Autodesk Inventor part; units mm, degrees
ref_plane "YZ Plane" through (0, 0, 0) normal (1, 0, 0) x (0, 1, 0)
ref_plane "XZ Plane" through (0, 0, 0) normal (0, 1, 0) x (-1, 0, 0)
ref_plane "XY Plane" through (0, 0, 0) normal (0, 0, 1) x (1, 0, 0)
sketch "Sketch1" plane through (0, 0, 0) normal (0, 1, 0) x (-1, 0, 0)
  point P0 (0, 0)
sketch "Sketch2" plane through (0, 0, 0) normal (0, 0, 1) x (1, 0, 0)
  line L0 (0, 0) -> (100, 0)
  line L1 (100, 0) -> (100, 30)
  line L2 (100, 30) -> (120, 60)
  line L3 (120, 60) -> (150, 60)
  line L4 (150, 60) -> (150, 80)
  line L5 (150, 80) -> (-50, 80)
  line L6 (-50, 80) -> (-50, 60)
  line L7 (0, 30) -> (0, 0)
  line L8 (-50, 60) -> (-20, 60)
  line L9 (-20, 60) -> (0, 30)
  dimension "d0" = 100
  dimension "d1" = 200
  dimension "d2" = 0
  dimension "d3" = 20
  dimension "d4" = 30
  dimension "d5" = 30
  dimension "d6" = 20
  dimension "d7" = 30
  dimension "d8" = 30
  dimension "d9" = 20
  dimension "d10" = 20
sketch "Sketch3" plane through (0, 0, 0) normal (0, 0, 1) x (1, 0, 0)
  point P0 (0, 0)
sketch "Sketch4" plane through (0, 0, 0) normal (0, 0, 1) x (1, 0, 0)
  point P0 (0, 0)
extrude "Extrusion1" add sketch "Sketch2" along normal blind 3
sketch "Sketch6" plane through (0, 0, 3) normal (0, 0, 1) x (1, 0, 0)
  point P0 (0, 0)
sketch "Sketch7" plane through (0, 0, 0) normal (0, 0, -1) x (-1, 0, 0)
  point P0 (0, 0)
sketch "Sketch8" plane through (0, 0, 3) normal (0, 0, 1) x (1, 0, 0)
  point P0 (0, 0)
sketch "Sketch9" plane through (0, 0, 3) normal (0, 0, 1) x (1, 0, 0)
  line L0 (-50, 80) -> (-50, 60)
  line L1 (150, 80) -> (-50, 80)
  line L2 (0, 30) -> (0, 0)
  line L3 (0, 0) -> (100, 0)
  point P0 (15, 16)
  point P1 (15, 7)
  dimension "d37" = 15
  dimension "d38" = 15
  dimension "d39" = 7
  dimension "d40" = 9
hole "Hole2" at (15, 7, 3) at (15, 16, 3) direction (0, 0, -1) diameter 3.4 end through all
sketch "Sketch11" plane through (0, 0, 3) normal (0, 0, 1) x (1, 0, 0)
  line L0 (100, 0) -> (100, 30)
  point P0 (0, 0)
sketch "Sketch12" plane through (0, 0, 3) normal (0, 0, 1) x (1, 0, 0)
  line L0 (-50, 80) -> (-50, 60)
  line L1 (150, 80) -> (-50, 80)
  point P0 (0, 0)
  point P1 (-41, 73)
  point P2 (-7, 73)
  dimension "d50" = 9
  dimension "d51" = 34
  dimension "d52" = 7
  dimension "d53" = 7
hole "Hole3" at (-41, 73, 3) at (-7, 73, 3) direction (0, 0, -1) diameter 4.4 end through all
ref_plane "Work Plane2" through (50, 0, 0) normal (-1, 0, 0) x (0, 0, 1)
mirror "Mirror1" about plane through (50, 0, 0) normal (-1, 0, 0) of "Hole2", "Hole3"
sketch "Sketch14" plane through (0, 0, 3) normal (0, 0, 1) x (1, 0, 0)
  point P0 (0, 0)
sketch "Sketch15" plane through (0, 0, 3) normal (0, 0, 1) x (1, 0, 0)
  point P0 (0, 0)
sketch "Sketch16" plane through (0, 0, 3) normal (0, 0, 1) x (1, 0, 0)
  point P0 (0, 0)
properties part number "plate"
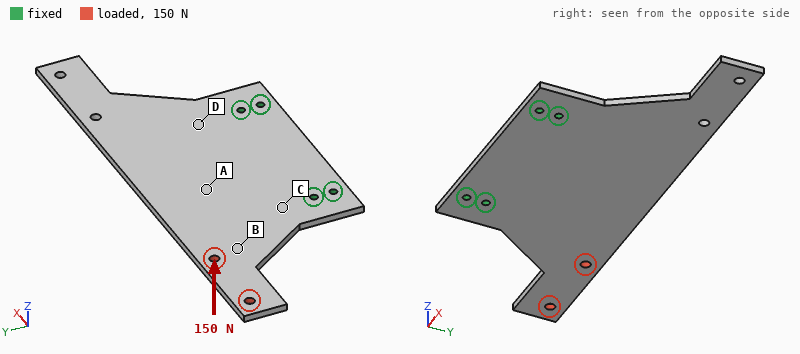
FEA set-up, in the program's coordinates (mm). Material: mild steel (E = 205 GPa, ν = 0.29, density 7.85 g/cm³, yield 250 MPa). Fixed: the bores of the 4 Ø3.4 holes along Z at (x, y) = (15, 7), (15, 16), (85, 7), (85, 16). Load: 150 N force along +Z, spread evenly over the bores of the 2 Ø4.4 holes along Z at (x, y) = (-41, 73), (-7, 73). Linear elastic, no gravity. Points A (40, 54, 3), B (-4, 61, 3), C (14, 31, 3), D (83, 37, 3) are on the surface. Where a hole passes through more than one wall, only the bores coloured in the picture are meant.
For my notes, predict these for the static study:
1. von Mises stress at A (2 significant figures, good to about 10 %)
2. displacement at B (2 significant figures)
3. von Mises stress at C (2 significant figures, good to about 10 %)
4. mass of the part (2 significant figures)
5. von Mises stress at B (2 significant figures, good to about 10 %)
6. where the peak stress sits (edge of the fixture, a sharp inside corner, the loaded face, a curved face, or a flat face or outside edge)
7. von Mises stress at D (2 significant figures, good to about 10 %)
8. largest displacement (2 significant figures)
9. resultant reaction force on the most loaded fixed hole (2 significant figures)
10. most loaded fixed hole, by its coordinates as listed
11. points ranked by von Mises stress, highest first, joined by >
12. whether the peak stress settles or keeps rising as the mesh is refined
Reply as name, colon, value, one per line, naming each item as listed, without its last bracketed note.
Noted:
von Mises stress at A: 49 MPa
displacement at B: 0.41 mm
von Mises stress at C: 91 MPa
mass of the part: 250 g
von Mises stress at B: 71 MPa
where the peak stress sits: edge of the fixture
von Mises stress at D: 19 MPa
largest displacement: 1.2 mm
resultant reaction force on the most loaded fixed hole: 560 N
most loaded fixed hole, by its coordinates as listed: (15, 16)
points ranked by von Mises stress, highest first, joined by >: C > B > A > D
whether the peak stress settles or keeps rising as the mesh is refined: keeps rising
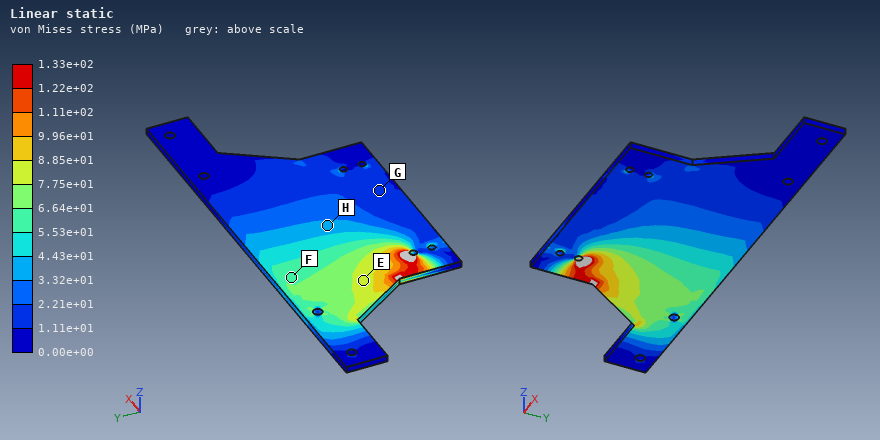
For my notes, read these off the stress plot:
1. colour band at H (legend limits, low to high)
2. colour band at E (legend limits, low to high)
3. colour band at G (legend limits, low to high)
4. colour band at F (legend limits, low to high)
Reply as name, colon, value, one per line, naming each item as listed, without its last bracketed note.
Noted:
colour band at H: 3.32e+01 to 4.43e+01 MPa
colour band at E: 7.75e+01 to 8.85e+01 MPa
colour band at G: 1.11e+01 to 2.21e+01 MPa
colour band at F: 5.53e+01 to 6.64e+01 MPa
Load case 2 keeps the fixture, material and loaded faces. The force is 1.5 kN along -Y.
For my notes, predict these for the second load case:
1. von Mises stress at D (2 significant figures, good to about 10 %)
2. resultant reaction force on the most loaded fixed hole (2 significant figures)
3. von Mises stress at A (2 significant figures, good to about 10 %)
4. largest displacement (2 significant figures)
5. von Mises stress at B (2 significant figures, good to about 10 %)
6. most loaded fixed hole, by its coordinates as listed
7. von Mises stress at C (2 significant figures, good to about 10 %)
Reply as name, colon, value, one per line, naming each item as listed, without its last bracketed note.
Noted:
von Mises stress at D: 8.3 MPa
resultant reaction force on the most loaded fixed hole: 1.6 kN
von Mises stress at A: 12 MPa
largest displacement: 66 µm
von Mises stress at B: 16 MPa
most loaded fixed hole, by its coordinates as listed: (15, 16)
von Mises stress at C: 24 MPa
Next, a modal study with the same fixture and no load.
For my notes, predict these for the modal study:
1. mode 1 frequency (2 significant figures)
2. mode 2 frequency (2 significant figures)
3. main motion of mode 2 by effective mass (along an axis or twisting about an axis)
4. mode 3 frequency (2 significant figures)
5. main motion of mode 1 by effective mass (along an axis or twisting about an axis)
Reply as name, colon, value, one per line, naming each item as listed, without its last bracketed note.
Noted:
mode 1 frequency: 380 Hz
mode 2 frequency: 420 Hz
main motion of mode 2 by effective mass: twisting about Y
mode 3 frequency: 710 Hz
main motion of mode 1 by effective mass: along Z
